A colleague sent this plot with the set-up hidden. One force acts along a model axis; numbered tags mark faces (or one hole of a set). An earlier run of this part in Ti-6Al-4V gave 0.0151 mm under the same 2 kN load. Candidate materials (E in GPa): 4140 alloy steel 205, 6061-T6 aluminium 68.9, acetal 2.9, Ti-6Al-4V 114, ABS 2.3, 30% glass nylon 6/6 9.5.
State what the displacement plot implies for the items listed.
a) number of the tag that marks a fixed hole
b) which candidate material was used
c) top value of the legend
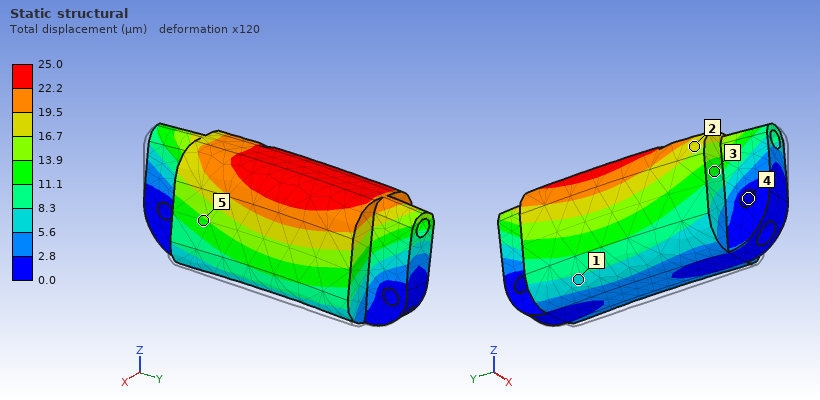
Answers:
4
6061-T6 aluminium
25.0 µm
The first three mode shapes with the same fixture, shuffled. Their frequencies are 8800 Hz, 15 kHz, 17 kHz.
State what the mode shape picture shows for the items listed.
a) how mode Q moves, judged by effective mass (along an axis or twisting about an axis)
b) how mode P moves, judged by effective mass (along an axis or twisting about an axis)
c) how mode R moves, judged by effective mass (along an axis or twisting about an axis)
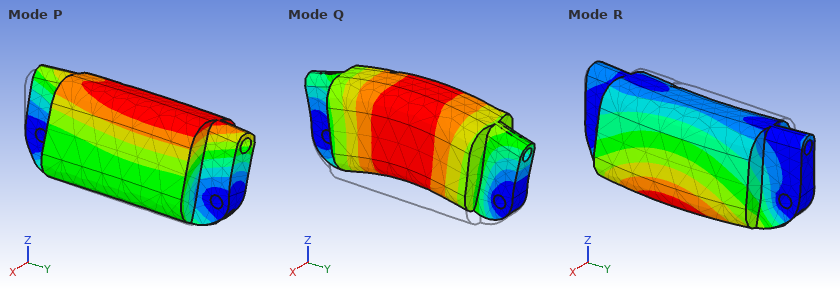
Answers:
along Z
along X
along X
